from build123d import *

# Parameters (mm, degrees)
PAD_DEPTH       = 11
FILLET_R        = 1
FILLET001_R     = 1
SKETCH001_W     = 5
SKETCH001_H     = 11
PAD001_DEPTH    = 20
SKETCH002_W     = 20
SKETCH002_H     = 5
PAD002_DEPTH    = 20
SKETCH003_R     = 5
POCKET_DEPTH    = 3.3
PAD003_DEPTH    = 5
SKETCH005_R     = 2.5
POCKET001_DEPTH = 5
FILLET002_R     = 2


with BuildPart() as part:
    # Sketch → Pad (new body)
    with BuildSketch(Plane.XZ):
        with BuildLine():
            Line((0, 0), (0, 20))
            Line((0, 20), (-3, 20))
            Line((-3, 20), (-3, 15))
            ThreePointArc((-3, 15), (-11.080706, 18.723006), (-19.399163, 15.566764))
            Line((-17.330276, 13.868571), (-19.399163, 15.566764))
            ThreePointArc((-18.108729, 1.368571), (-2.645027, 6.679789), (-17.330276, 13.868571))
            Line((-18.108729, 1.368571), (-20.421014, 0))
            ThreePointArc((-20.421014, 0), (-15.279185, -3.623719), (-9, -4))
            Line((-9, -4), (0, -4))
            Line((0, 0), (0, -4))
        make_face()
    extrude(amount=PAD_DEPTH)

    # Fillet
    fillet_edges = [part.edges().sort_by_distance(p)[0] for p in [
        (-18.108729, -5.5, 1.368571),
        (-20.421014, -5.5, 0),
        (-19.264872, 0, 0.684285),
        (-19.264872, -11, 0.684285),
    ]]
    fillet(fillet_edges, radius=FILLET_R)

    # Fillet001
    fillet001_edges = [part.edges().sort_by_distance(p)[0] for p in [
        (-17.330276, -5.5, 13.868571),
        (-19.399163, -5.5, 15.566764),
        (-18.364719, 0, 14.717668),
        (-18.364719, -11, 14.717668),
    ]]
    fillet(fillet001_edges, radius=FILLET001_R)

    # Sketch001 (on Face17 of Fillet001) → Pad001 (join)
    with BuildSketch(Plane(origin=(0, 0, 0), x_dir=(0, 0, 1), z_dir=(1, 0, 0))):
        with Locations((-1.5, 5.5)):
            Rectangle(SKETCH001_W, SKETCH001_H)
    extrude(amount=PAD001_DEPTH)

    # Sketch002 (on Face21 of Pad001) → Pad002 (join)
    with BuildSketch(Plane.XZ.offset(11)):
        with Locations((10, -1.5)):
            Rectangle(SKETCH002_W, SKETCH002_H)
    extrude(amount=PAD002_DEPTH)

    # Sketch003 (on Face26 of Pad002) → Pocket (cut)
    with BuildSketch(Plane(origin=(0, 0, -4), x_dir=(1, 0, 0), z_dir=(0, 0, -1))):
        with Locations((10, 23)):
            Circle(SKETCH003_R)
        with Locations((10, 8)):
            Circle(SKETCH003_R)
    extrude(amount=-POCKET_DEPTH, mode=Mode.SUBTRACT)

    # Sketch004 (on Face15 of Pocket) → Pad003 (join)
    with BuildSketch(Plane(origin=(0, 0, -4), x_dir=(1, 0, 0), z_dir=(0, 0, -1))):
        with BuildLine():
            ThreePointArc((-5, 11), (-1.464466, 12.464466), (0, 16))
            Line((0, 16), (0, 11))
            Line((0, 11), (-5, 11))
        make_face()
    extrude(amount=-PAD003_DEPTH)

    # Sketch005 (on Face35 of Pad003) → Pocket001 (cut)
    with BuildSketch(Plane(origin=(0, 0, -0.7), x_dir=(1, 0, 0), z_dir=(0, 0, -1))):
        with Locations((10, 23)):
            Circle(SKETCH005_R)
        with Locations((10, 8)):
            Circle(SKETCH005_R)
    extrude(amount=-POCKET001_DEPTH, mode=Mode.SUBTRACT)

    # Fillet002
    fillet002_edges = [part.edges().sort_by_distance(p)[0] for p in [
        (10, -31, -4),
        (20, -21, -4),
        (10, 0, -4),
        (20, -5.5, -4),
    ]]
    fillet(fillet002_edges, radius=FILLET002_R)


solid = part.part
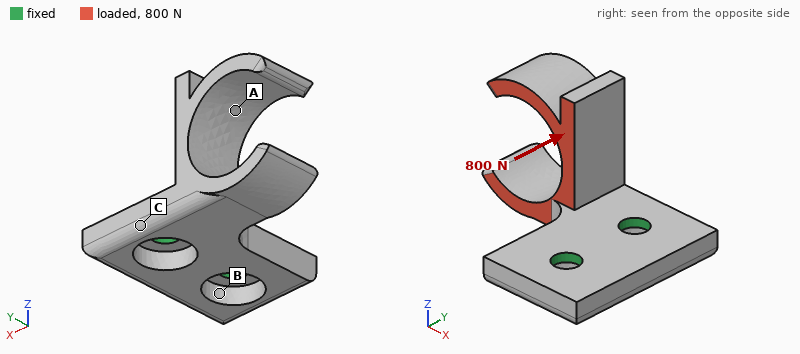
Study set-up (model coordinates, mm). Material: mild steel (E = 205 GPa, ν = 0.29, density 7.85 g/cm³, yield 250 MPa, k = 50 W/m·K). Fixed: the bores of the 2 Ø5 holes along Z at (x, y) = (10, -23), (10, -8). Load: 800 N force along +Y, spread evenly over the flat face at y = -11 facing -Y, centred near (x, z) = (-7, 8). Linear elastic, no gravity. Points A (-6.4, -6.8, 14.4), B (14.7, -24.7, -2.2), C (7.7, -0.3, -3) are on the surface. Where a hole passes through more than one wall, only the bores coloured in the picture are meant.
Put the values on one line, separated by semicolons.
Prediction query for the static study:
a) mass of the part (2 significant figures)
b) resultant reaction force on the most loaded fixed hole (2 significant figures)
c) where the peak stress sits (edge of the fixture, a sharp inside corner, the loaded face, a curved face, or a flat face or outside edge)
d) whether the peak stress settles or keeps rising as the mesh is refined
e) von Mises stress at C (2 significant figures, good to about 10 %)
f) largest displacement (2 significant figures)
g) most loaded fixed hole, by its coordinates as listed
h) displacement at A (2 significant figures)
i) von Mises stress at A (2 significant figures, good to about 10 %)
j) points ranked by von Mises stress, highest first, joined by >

35 g; 1.0 kN; edge of the fixture; keeps rising; 120 MPa; 0.12 mm; (10, -8); 0.068 mm; 48 MPa; C > A > B
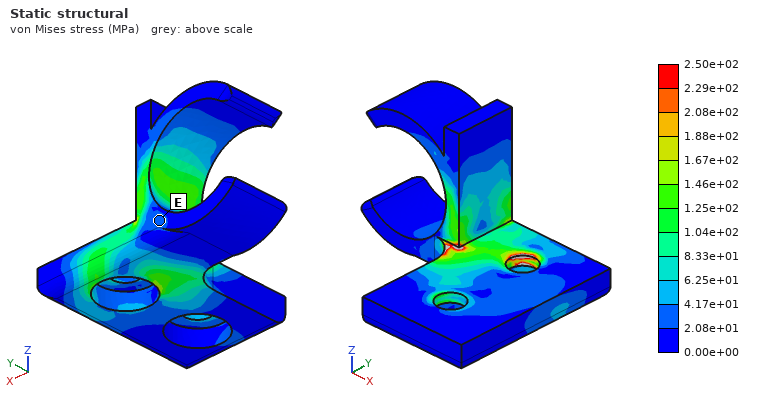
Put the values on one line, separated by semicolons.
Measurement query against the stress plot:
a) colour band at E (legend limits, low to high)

2.08e+01 to 4.17e+01 MPa
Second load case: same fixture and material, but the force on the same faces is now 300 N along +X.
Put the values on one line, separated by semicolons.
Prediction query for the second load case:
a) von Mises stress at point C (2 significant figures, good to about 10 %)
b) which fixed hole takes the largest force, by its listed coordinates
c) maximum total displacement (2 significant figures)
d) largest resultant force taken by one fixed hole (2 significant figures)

41 MPa; (10, -8); 0.12 mm; 270 N
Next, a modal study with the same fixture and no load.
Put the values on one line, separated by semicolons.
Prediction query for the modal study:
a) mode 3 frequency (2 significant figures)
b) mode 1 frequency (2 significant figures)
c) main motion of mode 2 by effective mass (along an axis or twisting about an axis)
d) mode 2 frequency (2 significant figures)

5800 Hz; 2300 Hz; along Y; 4400 Hz
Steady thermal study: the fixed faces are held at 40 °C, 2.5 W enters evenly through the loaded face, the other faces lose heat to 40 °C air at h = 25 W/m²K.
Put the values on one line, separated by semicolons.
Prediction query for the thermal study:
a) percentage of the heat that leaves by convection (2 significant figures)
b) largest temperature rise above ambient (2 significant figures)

22 %; 20 K
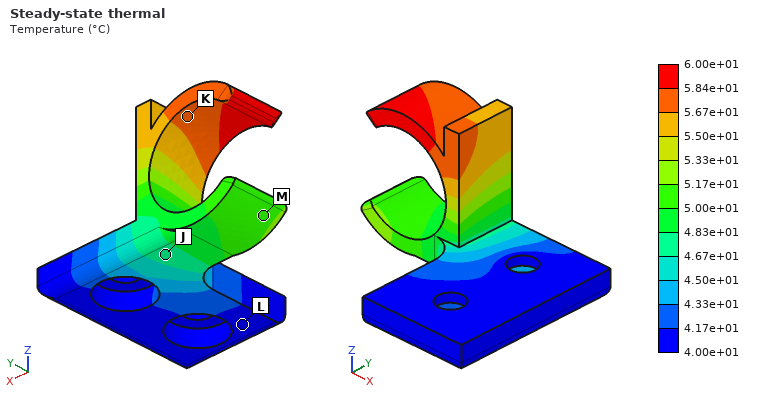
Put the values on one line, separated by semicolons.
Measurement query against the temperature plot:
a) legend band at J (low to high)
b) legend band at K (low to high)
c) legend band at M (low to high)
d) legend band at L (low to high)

4.67e+01 to 4.83e+01 °C; 5.67e+01 to 5.84e+01 °C; 5.00e+01 to 5.17e+01 °C; 4.00e+01 to 4.17e+01 °C
